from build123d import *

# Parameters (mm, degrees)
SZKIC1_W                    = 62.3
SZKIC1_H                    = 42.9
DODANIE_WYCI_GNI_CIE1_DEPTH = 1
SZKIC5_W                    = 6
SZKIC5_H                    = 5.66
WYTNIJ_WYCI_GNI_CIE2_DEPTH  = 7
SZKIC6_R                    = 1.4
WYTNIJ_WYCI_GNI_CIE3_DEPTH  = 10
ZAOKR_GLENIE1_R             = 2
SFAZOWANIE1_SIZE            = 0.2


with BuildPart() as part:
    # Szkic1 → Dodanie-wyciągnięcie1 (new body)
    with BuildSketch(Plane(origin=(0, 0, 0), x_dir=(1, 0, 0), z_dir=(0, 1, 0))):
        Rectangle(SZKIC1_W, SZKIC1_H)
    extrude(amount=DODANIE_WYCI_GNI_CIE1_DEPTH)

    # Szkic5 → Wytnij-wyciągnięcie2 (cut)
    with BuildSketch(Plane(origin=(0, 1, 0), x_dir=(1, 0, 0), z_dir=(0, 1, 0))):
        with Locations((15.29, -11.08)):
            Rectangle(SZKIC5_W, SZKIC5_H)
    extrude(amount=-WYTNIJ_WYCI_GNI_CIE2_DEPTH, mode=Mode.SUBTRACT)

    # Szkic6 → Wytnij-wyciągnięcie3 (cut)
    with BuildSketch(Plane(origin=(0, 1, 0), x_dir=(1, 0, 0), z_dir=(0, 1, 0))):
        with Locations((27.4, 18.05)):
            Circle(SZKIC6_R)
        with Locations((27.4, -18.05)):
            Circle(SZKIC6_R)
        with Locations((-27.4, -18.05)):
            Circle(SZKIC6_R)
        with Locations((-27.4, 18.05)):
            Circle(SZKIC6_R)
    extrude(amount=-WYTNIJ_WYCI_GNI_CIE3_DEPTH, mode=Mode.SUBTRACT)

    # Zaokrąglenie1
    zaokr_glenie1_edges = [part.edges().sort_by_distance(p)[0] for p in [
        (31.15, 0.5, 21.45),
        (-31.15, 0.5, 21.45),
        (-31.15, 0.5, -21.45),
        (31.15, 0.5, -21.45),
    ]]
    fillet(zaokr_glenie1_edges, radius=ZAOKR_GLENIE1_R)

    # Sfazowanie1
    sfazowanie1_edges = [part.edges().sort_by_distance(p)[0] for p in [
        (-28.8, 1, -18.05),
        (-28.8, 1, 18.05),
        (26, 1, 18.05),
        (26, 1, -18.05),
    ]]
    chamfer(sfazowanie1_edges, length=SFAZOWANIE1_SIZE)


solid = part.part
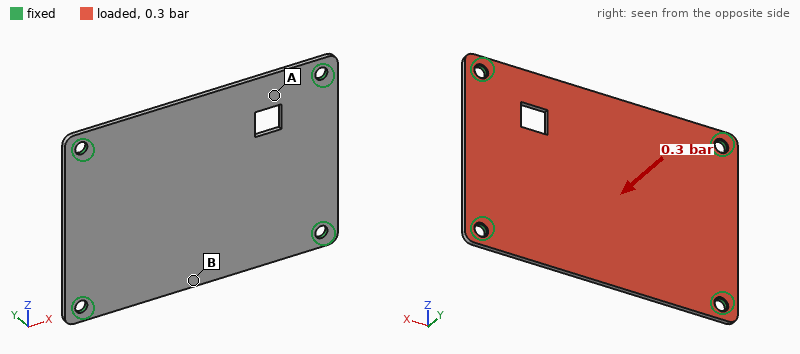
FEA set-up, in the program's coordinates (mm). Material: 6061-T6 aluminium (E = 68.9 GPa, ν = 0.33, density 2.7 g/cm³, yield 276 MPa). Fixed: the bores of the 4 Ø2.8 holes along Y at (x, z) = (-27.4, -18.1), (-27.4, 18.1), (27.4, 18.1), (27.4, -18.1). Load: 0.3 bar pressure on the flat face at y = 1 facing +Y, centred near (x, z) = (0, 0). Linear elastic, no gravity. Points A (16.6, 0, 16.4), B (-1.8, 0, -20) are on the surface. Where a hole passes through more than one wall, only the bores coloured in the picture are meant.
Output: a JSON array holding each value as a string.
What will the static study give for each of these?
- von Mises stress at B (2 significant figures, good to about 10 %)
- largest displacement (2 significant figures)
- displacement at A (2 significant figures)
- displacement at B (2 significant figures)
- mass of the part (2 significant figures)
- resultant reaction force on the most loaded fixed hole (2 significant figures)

["28 MPa", "0.17 mm", "0.066 mm", "0.15 mm", "7.0 g", "20 N"]
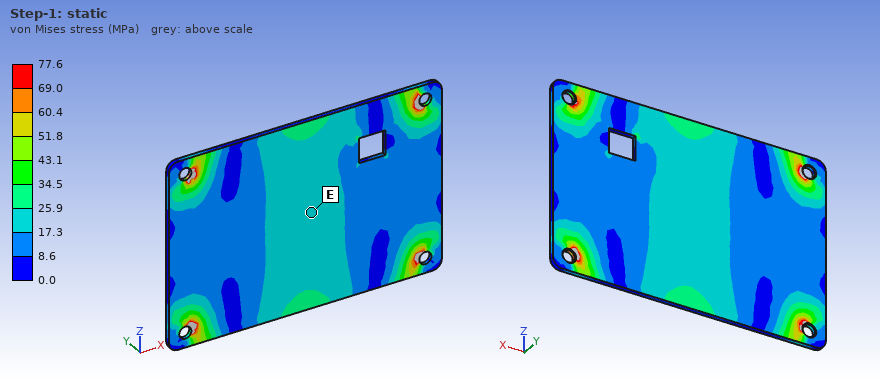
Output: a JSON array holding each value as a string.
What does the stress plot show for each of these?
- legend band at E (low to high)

["17.3 to 25.9 MPa"]
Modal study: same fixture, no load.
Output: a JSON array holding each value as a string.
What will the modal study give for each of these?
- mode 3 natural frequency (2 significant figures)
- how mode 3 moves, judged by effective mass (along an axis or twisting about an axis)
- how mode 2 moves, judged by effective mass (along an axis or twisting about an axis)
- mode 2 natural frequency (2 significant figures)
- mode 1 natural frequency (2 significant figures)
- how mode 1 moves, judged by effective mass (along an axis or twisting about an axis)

["3600 Hz", "twisting about Z", "twisting about X", "2300 Hz", "1500 Hz", "along Y"]
